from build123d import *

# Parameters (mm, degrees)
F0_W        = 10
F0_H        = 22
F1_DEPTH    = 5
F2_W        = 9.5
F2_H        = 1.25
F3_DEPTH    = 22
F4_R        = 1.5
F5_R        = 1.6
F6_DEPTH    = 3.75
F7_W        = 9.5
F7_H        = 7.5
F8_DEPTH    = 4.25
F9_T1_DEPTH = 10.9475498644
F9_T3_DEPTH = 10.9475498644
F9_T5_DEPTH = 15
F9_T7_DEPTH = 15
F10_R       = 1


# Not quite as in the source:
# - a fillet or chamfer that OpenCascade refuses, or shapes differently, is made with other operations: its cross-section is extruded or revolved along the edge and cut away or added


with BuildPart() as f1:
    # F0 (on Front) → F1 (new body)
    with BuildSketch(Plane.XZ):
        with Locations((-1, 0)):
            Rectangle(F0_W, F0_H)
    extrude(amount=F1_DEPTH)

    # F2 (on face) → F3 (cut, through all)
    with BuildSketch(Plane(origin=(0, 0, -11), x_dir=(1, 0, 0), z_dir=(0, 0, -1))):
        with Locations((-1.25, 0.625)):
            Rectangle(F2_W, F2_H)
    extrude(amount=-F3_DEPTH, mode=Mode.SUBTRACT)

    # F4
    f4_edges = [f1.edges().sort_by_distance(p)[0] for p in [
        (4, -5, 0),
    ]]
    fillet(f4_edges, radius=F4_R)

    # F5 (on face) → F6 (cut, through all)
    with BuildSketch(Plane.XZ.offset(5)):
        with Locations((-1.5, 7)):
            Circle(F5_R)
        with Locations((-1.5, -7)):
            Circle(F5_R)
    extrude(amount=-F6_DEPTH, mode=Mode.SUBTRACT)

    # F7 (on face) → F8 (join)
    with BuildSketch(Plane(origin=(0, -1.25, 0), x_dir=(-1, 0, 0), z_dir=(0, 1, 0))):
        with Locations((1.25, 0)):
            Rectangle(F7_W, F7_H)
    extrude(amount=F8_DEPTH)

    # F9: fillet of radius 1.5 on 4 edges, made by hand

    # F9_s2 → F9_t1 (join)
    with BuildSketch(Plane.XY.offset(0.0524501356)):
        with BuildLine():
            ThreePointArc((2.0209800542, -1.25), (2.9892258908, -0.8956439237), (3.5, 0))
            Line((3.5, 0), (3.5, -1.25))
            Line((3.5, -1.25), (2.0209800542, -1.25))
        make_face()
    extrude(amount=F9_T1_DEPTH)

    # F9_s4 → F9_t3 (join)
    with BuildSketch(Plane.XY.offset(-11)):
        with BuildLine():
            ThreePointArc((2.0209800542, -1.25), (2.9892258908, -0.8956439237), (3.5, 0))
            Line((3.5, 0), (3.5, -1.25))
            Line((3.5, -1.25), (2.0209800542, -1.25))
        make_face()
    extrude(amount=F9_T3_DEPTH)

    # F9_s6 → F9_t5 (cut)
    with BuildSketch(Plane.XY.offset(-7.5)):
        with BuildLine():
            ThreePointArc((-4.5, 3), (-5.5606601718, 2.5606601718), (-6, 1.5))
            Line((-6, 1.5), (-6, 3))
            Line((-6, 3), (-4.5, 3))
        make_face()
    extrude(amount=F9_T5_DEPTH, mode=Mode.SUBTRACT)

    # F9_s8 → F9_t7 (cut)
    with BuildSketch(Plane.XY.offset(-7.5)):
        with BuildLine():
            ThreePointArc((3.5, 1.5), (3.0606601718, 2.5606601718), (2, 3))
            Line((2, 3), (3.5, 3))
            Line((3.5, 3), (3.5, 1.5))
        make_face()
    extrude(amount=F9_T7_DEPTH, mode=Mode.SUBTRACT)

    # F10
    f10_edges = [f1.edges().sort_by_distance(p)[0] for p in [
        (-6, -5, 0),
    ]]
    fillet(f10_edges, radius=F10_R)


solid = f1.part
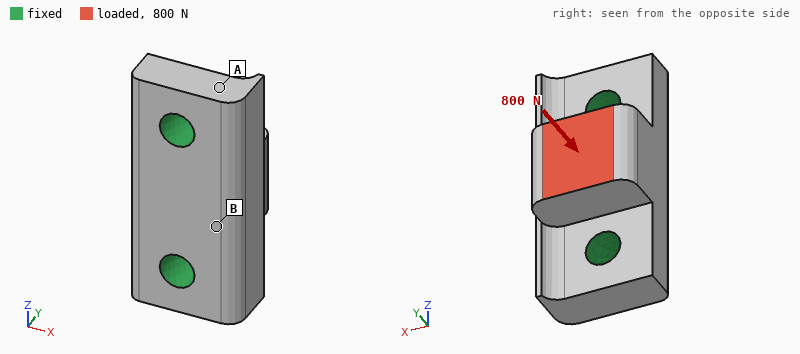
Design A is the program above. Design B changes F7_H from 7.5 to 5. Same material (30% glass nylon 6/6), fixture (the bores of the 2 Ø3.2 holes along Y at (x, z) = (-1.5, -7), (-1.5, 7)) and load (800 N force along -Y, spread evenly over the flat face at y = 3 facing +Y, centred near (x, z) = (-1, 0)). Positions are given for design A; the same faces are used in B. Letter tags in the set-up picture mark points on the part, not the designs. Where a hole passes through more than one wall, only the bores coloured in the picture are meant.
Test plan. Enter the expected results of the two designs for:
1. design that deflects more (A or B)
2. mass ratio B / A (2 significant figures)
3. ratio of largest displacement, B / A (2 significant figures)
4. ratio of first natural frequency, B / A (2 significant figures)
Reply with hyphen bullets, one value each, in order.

- B
- 0.91
- 1.5
- 1.0
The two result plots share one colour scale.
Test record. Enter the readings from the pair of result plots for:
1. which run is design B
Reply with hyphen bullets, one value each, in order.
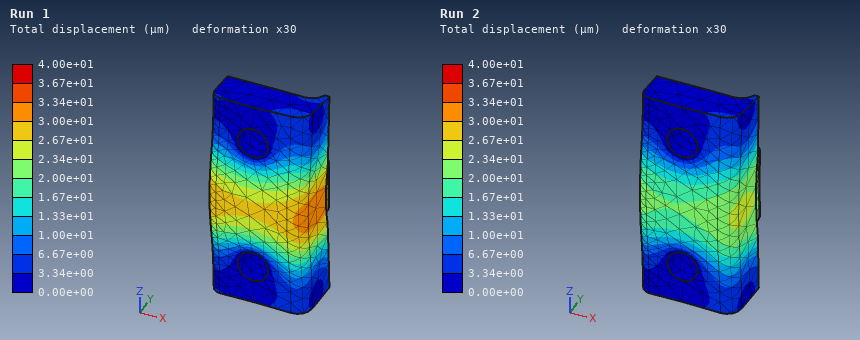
- Run 1
